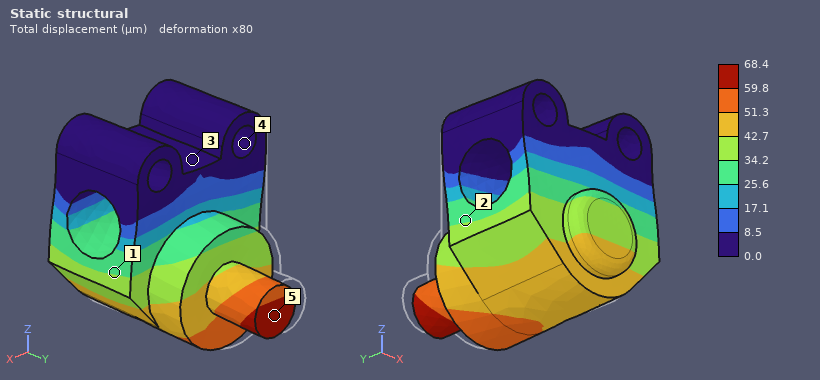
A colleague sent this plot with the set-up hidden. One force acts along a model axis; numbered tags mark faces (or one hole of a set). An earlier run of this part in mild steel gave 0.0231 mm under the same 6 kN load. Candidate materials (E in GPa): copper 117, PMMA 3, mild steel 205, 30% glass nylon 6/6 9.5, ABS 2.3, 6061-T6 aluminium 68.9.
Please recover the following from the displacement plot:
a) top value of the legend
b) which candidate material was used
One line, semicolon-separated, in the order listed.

68.4 µm; 6061-T6 aluminium
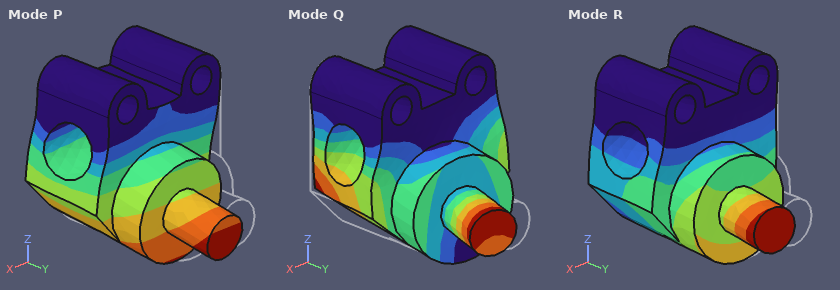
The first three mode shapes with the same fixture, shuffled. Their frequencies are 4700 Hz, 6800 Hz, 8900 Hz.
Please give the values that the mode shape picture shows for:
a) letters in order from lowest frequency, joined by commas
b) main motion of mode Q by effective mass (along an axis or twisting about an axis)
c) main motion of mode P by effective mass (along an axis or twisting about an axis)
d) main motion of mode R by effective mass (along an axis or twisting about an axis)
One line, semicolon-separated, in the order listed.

P, R, Q; along X; along Y; along X
